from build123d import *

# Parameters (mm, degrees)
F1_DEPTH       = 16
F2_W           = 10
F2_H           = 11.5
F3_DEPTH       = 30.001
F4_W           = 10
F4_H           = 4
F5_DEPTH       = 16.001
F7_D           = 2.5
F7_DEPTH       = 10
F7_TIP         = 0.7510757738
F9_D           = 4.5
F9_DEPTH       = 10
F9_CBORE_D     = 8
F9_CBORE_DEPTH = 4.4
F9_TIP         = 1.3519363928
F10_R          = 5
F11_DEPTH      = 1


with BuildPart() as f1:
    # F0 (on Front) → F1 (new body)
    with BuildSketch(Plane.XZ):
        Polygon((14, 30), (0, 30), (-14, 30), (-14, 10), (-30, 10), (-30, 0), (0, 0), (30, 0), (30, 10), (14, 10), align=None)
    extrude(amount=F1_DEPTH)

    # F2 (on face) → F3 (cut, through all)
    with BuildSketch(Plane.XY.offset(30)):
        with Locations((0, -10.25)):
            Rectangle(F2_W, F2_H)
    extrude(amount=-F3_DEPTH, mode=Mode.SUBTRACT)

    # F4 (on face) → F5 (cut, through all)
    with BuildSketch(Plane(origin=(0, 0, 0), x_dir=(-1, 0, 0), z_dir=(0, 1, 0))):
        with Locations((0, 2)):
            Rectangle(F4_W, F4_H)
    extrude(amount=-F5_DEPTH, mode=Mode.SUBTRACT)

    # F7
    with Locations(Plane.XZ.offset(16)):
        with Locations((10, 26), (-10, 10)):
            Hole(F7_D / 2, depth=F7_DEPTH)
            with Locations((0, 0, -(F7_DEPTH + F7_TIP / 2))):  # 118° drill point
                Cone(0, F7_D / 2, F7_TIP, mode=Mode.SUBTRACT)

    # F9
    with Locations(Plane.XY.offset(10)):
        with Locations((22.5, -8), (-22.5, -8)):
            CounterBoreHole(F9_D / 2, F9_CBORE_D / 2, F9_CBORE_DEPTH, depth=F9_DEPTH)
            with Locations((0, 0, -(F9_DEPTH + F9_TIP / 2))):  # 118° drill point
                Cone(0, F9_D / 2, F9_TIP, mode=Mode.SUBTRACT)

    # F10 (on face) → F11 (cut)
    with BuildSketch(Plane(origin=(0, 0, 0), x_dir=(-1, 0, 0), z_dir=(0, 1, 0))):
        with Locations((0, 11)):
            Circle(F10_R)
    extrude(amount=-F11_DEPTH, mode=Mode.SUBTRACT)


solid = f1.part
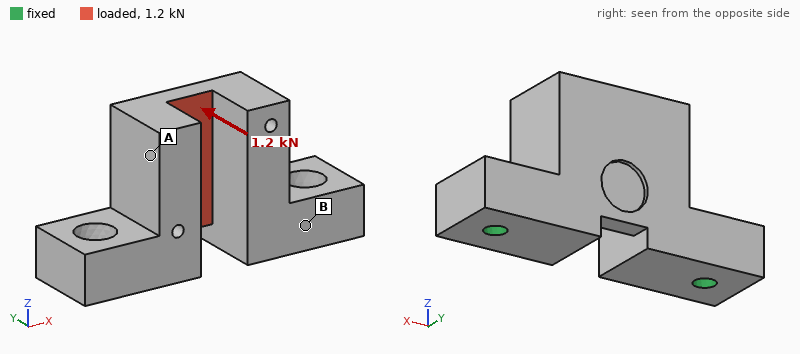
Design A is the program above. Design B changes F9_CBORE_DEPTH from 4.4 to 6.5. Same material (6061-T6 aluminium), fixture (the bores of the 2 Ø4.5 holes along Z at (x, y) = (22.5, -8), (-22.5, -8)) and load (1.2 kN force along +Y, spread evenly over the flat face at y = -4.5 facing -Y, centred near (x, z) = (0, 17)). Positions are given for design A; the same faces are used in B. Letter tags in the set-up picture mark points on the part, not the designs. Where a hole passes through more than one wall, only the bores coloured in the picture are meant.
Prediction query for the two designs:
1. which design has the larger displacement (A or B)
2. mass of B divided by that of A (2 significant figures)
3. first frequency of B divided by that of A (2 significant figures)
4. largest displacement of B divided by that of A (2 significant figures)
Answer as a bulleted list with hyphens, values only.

- B
- 0.99
- 0.75
- 1.7
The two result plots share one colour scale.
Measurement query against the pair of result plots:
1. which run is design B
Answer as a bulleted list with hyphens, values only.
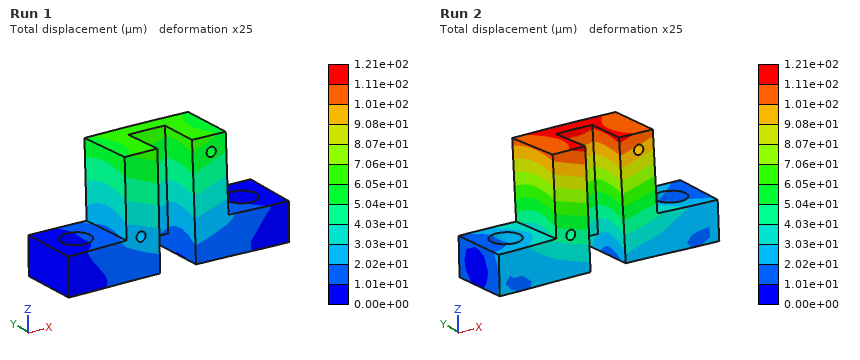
- Run 2
